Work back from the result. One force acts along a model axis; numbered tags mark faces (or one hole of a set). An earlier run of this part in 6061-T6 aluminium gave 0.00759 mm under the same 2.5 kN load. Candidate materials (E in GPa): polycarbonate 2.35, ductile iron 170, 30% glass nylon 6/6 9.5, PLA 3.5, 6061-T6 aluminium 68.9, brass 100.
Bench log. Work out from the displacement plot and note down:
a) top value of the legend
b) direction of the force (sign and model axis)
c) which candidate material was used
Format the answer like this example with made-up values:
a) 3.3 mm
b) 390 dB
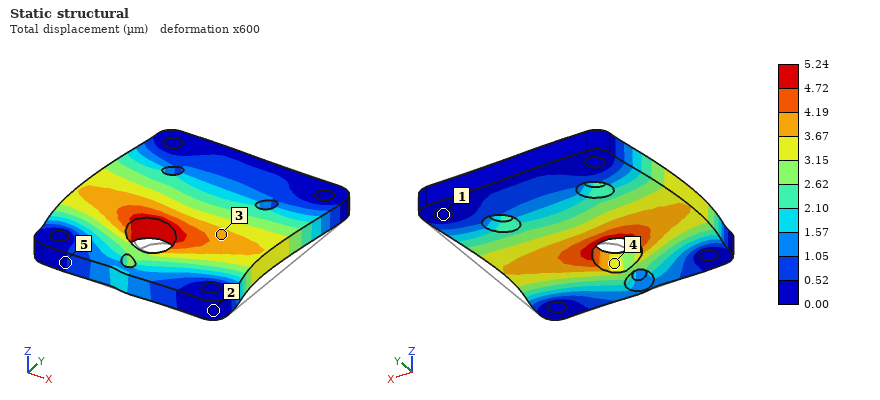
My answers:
a) 5.24 µm
b) -X
c) brass
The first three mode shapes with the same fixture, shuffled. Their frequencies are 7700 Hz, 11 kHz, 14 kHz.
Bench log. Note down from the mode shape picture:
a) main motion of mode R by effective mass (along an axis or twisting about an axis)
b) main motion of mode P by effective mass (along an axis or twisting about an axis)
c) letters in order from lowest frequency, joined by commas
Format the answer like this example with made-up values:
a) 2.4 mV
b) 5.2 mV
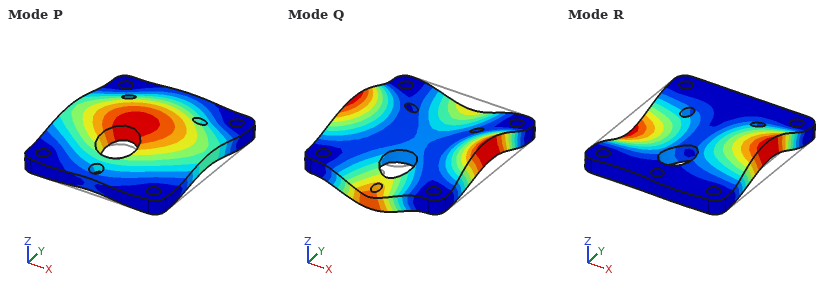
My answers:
a) twisting about Y
b) along Z
c) P, R, Q
